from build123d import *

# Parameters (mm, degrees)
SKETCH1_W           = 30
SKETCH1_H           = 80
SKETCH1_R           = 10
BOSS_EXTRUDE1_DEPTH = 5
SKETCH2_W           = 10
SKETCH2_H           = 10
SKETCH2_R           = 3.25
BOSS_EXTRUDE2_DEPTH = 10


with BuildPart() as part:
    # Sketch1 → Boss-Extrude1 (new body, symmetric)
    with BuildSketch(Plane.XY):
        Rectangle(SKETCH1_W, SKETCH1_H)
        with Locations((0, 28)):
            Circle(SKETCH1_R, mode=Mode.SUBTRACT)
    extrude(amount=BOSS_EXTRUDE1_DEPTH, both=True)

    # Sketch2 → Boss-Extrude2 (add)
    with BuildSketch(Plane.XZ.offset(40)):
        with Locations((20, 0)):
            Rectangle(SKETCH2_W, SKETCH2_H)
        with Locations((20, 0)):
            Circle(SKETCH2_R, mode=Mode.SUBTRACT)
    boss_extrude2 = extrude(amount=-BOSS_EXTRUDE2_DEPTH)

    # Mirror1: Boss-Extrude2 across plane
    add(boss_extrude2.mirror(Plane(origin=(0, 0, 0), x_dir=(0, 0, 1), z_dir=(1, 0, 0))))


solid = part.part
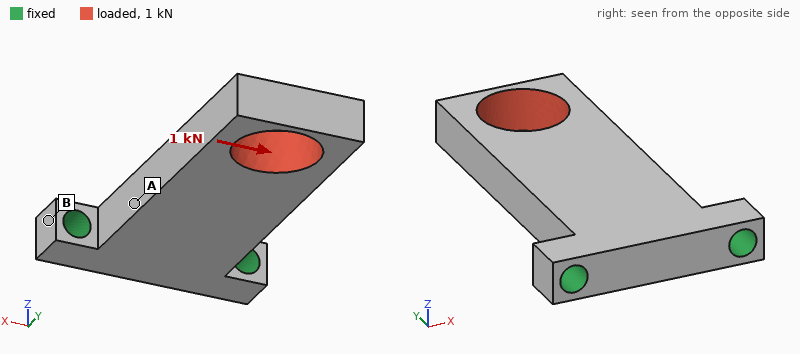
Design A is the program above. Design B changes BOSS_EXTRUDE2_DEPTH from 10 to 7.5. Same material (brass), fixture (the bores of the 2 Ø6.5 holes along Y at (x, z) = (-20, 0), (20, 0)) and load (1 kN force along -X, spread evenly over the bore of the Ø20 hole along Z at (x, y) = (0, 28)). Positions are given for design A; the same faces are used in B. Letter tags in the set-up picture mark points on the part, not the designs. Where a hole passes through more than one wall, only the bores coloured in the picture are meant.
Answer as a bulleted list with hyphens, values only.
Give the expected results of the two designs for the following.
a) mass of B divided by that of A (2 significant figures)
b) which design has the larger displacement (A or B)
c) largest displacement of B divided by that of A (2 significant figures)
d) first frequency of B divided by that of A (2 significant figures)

- 0.98
- B
- 1.1
- 0.85
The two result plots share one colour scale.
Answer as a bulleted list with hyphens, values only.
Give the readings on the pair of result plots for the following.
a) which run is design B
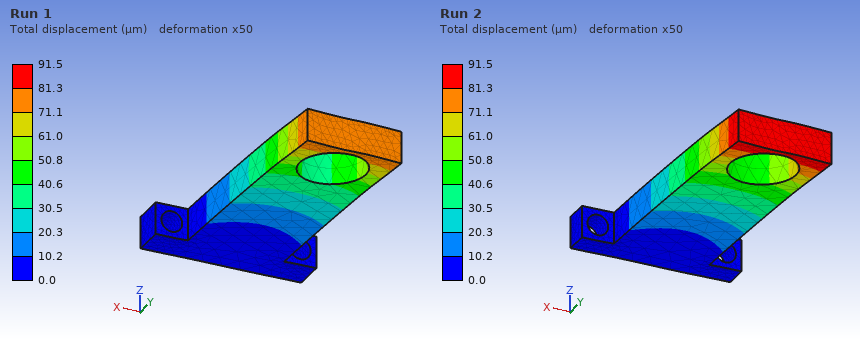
- Run 2
